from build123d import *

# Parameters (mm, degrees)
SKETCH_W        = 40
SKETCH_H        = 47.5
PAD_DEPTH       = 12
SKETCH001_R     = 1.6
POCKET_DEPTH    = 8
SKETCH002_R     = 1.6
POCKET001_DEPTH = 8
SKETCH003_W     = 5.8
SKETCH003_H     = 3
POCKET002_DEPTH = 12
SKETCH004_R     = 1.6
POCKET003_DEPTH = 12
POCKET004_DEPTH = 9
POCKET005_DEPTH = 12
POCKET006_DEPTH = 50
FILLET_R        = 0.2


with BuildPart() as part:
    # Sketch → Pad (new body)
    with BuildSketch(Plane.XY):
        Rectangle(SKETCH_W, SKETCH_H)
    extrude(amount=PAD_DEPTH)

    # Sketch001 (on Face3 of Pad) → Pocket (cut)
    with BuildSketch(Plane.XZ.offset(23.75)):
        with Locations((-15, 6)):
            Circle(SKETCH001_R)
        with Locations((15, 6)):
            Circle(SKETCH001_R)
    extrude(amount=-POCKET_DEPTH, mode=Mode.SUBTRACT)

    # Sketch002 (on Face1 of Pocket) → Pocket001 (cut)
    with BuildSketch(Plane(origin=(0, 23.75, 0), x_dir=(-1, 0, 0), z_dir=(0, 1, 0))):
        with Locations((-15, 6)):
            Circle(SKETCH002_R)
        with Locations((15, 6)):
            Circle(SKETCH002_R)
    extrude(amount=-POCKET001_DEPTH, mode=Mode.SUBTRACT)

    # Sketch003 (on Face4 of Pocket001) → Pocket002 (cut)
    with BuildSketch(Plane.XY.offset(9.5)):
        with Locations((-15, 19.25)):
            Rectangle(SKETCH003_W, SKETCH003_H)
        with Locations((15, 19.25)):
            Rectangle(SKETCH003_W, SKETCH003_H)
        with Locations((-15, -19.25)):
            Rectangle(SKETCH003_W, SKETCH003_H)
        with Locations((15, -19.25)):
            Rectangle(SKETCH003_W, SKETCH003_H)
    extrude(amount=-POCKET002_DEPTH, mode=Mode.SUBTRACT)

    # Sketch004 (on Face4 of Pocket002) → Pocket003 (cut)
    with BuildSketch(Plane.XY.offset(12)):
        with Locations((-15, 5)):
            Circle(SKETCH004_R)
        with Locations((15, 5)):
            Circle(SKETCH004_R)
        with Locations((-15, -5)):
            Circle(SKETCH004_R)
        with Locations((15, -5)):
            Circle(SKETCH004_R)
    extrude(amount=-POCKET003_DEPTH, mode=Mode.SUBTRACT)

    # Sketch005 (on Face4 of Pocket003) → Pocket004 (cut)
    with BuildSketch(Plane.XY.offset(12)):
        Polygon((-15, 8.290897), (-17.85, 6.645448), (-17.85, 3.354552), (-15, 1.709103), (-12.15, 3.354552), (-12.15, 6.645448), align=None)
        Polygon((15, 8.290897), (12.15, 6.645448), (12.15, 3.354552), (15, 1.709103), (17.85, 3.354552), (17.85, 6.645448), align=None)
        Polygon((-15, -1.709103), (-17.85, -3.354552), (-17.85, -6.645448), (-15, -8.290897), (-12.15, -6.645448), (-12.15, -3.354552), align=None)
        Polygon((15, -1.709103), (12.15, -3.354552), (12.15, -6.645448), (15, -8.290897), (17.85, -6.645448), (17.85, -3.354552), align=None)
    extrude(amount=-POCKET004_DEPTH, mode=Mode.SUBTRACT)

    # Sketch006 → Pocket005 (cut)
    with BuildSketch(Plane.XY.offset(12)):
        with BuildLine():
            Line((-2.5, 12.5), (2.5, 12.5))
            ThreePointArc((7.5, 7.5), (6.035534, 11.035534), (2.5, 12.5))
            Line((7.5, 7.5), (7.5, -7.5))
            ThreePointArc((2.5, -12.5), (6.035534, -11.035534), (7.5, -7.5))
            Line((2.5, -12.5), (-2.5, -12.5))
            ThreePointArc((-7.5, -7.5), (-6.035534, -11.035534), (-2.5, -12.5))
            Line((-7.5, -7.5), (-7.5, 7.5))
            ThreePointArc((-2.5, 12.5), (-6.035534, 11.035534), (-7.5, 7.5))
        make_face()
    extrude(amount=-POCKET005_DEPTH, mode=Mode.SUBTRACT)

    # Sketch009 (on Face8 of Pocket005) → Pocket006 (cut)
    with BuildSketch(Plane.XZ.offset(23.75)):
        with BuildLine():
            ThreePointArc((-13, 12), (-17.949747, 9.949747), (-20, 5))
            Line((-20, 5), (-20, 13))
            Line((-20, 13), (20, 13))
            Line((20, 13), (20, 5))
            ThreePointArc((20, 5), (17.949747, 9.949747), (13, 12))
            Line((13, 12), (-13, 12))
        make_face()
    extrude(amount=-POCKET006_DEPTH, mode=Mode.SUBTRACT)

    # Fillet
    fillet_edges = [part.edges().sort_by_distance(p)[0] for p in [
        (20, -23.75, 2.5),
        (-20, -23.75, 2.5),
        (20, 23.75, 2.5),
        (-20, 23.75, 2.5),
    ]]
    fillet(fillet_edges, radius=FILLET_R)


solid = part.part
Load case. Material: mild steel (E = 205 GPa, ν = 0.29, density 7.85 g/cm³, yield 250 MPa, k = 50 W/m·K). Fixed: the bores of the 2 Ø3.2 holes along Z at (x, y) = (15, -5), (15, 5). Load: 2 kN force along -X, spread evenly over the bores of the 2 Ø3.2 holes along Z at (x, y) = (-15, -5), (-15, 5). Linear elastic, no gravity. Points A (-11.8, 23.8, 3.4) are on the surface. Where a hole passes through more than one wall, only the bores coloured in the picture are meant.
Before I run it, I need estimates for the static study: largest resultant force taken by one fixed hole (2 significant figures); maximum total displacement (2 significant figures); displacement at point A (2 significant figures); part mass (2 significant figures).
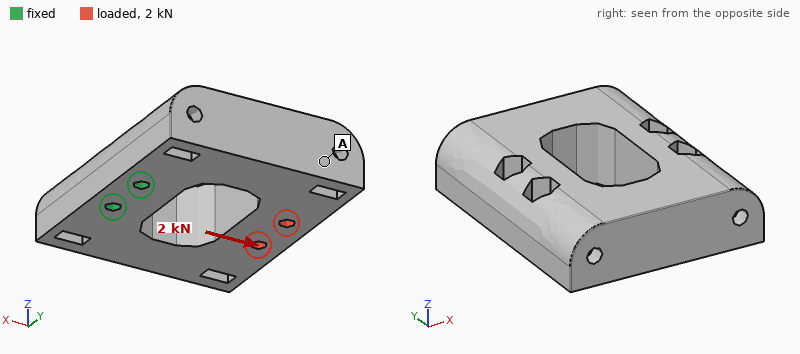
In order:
1.0 kN
17 µm
6.6 µm
120 g
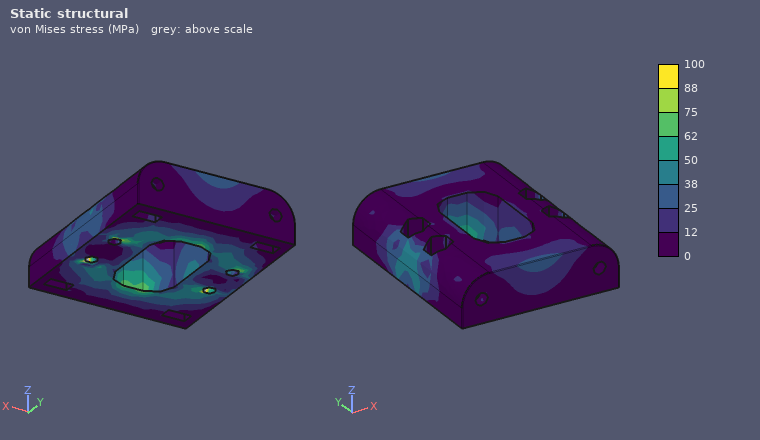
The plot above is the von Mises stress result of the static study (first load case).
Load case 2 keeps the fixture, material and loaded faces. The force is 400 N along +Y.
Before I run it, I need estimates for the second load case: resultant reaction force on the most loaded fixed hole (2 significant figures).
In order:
910 N
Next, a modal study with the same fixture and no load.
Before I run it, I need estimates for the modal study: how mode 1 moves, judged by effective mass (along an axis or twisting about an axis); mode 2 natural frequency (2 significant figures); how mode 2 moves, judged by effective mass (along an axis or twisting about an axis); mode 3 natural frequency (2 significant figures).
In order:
along Z
3700 Hz
along Y
4600 Hz
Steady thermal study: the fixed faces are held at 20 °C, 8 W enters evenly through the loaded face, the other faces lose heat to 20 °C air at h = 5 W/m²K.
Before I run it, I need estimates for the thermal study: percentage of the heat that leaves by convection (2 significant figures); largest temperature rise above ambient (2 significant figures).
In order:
7.1 %
35 K
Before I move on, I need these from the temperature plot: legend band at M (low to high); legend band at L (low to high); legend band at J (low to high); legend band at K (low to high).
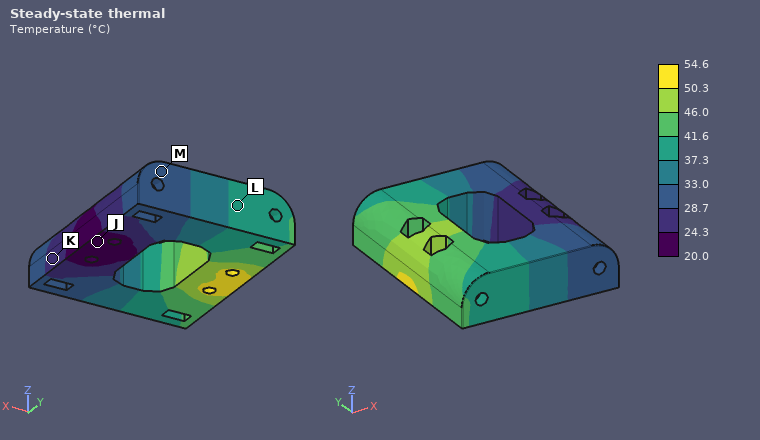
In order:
28.7 to 33.0 °C
37.3 to 41.6 °C
20.0 to 24.3 °C
24.3 to 28.7 °C
